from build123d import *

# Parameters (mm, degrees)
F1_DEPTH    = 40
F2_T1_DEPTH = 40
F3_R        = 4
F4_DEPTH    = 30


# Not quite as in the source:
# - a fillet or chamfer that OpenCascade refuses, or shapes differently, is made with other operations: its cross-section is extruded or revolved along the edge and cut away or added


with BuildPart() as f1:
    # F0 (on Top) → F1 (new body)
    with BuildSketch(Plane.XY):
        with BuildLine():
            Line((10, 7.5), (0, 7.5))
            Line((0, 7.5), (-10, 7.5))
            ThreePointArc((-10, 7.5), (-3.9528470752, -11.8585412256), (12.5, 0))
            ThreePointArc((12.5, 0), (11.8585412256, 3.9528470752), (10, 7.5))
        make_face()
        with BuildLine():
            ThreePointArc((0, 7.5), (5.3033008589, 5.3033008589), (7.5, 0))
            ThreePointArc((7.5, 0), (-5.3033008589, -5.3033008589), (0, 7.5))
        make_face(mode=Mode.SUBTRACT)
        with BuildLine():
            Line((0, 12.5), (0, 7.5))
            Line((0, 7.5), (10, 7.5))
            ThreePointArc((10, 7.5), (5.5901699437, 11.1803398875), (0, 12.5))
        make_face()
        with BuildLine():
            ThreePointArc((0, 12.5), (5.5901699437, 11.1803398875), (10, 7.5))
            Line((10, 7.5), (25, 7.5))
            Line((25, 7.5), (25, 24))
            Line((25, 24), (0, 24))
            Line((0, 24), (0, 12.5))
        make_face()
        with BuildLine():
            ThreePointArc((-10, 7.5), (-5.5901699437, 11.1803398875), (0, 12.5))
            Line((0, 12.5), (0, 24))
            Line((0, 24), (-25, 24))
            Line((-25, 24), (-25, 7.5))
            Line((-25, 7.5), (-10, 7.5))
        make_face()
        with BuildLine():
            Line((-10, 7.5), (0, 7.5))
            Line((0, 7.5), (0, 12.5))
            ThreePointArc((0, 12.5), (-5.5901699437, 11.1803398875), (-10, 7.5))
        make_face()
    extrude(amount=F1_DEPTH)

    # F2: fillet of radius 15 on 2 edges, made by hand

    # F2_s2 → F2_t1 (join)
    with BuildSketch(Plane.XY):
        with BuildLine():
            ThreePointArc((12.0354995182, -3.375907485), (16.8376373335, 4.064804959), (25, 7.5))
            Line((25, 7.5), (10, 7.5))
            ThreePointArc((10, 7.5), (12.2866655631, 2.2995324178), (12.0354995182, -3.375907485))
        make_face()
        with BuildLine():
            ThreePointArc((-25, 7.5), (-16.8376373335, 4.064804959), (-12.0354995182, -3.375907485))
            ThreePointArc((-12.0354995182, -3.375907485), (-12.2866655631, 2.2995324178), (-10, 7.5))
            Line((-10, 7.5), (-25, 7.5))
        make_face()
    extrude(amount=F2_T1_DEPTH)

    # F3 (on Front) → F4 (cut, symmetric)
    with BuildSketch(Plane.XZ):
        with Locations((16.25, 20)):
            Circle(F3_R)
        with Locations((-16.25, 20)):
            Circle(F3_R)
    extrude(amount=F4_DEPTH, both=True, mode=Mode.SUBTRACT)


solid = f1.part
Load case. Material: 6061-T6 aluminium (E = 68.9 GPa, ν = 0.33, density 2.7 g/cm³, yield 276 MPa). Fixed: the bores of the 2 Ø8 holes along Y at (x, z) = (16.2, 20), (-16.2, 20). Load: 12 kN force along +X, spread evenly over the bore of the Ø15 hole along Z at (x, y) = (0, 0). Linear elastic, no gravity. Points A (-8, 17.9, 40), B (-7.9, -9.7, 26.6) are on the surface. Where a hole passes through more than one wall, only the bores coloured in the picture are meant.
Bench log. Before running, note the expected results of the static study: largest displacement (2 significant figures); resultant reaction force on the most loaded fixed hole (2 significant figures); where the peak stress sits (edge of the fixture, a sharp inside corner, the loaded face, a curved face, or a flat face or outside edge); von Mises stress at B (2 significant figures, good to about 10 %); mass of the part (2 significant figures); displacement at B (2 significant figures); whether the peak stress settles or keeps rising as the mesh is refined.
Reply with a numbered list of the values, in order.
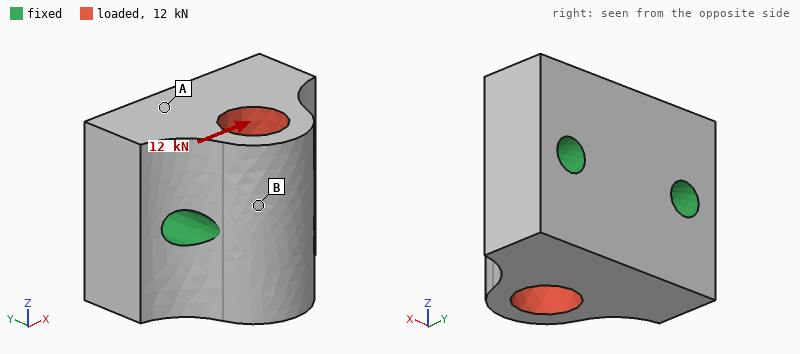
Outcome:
1. 14 µm
2. 6.5 kN
3. edge of the fixture
4. 18 MPa
5. 120 g
6. 12 µm
7. keeps rising
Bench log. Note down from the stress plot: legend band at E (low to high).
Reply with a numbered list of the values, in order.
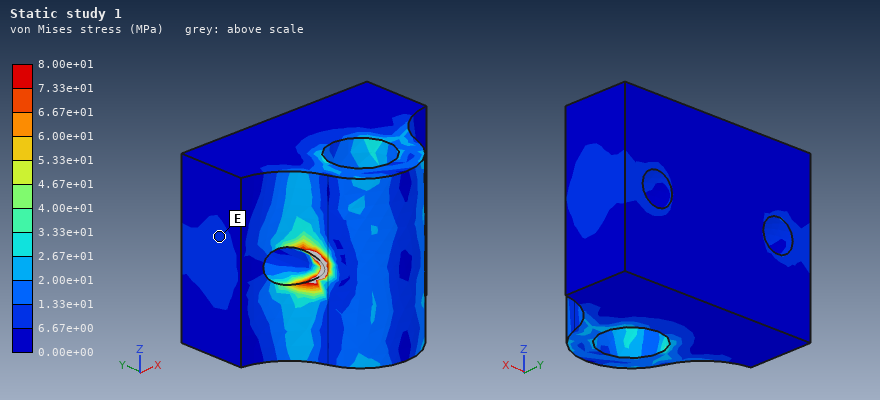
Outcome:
1. 6.67e+00 to 1.33e+01 MPa
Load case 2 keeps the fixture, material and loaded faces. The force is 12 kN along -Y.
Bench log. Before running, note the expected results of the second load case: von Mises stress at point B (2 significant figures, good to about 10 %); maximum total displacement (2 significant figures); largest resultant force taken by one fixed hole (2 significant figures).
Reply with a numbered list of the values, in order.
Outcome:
1. 13 MPa
2. 8.5 µm
3. 6.1 kN
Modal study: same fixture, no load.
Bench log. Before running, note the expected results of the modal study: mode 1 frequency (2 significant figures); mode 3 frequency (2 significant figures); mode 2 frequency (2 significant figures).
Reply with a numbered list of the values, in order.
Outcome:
1. 22 kHz
2. 29 kHz
3. 28 kHz
